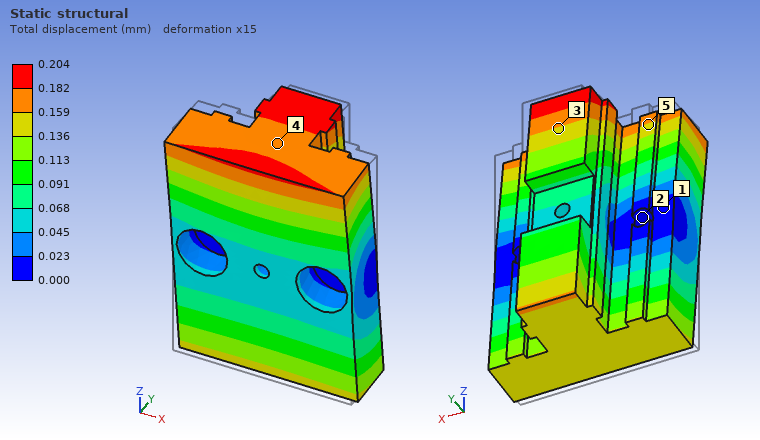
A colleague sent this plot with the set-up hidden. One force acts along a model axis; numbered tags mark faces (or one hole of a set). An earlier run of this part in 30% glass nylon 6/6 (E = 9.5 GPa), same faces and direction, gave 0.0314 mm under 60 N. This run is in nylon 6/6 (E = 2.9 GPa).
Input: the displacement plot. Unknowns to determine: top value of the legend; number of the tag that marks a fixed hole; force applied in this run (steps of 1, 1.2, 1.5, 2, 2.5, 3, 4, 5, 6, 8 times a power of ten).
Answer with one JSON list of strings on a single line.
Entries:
["0.204 mm", "2", "120 N"]
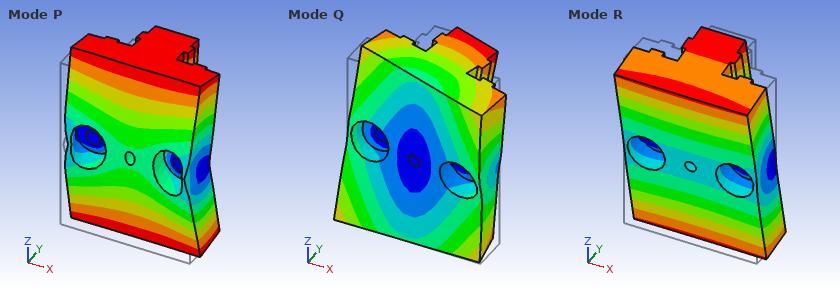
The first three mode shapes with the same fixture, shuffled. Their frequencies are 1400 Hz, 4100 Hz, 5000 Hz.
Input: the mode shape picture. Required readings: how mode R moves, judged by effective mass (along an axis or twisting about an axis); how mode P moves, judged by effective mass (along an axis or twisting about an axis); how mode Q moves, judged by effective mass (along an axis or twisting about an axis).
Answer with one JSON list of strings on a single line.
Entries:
["twisting about X", "along Y", "twisting about Y"]
